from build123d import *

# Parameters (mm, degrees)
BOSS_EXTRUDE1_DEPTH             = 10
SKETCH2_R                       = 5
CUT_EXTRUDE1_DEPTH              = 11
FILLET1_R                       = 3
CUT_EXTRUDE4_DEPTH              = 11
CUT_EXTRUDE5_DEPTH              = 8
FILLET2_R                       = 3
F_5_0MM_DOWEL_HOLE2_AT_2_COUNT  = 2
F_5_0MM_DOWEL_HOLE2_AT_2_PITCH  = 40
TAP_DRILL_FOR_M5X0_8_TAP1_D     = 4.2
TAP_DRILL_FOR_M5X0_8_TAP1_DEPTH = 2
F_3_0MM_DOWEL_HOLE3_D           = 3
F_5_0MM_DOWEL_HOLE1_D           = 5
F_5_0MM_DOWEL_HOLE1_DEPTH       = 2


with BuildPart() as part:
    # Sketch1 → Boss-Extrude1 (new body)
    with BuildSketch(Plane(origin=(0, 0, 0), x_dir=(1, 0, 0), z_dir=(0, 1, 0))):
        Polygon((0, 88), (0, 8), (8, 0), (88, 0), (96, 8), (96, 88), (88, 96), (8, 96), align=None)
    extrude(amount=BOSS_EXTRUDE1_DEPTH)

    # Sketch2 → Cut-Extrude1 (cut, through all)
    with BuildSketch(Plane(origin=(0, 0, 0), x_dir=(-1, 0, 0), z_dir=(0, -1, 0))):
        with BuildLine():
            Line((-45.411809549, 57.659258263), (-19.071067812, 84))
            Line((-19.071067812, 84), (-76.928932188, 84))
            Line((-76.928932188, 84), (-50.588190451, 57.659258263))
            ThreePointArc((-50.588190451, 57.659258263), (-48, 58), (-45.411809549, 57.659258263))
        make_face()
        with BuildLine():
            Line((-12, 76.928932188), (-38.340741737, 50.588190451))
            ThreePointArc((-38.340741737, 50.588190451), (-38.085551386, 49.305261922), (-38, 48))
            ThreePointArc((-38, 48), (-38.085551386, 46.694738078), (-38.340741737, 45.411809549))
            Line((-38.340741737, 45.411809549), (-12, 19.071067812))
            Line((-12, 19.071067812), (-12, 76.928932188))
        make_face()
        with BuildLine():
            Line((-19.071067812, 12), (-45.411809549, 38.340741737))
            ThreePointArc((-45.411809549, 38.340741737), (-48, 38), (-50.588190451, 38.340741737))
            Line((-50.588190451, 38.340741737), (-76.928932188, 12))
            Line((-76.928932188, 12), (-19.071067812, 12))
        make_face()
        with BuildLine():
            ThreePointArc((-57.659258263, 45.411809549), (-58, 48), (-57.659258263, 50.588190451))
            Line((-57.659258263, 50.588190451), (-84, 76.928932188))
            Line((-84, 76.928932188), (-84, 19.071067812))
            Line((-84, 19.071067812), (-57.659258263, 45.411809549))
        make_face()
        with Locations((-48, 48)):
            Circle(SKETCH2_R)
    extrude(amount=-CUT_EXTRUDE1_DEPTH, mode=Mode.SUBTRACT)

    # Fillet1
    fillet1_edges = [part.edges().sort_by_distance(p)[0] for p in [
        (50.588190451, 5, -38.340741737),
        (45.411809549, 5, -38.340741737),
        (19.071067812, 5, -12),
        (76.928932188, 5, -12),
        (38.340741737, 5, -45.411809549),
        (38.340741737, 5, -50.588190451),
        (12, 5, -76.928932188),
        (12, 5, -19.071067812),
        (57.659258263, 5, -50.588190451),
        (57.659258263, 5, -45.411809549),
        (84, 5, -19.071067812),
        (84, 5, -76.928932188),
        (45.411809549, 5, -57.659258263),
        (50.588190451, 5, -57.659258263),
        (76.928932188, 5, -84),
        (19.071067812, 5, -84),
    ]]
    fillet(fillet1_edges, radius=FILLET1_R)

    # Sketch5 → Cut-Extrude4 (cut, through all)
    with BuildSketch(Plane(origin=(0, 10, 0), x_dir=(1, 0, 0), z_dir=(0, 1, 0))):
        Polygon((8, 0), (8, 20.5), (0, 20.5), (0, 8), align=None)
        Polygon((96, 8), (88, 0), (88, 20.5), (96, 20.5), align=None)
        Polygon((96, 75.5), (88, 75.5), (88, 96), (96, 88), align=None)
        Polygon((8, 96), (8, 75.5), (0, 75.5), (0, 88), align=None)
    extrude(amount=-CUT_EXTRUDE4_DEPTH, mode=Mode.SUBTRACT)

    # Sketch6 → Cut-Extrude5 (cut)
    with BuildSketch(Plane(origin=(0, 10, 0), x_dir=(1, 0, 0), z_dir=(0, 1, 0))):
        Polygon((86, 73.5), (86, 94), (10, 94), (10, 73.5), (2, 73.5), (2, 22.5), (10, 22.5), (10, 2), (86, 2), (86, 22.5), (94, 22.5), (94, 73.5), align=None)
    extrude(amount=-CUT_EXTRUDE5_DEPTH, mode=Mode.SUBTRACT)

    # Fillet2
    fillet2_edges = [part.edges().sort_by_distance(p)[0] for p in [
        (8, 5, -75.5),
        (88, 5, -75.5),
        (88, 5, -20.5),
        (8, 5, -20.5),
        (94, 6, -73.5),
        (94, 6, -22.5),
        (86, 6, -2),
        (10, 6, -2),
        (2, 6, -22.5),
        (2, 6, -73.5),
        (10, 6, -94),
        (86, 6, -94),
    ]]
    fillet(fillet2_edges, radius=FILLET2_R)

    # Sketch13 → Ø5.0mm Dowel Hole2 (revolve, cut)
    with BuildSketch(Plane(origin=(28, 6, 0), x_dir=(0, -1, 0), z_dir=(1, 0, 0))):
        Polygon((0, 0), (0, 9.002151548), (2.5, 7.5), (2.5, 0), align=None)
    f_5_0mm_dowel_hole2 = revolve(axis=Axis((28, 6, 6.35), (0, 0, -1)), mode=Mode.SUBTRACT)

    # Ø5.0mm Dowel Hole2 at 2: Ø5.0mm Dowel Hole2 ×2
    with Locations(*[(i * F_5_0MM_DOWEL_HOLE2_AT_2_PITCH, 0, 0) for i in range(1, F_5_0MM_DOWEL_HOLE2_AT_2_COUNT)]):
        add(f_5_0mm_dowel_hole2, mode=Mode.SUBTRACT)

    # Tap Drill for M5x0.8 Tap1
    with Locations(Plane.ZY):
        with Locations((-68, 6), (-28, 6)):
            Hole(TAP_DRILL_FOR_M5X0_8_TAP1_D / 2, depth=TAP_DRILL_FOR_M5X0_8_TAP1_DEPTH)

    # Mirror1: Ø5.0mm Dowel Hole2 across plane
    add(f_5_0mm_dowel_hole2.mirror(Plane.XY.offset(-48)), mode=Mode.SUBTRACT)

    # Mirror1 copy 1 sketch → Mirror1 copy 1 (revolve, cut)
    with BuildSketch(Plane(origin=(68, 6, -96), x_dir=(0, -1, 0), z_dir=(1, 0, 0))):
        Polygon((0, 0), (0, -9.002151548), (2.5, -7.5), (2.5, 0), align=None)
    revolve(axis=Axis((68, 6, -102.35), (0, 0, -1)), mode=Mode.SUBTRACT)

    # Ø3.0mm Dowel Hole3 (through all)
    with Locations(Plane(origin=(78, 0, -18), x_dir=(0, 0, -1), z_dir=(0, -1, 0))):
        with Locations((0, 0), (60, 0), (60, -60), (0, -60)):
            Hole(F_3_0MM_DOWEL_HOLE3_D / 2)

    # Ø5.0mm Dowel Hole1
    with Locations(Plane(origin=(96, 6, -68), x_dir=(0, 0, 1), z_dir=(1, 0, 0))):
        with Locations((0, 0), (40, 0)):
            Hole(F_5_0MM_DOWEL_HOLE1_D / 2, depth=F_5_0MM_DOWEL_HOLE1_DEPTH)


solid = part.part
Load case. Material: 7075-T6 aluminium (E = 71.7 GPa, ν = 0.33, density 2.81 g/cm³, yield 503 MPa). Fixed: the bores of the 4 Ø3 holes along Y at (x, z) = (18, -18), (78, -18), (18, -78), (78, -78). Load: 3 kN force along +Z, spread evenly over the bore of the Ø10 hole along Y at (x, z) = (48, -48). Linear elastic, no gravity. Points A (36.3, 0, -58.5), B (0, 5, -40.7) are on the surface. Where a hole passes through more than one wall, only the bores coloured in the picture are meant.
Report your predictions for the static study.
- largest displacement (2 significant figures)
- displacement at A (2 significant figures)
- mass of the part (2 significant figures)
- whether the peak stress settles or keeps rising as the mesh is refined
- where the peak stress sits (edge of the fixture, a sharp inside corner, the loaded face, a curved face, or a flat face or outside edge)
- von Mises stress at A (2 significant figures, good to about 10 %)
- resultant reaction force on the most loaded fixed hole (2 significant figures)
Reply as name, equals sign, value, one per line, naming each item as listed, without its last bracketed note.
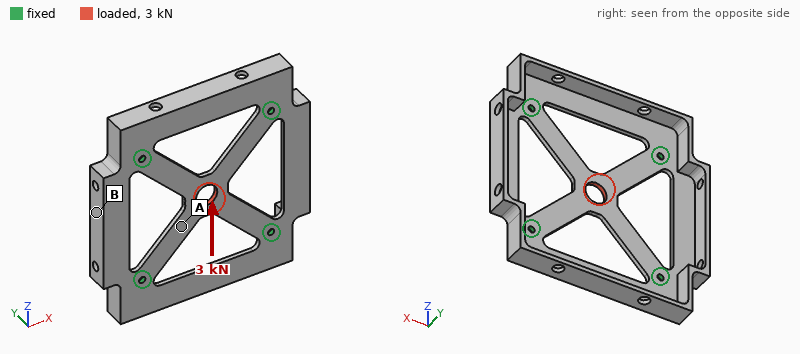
largest displacement = 43 µm
displacement at A = 28 µm
mass of the part = 46 g
whether the peak stress settles or keeps rising as the mesh is refined = keeps rising
where the peak stress sits = edge of the fixture
von Mises stress at A = 51 MPa
resultant reaction force on the most loaded fixed hole = 980 N
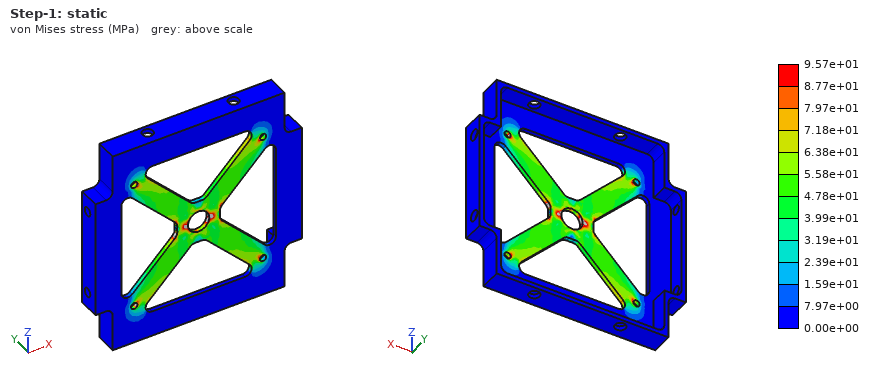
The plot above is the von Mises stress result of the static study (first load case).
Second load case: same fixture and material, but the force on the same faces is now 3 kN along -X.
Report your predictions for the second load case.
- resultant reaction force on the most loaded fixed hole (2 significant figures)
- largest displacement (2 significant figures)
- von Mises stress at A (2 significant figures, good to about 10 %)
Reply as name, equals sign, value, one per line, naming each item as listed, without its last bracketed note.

resultant reaction force on the most loaded fixed hole = 980 N
largest displacement = 43 µm
von Mises stress at A = 49 MPa
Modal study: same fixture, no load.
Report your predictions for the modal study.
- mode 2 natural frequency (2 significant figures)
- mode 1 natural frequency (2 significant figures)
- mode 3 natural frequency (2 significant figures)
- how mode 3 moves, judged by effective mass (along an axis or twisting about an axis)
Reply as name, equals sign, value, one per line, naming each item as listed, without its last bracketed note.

mode 2 natural frequency = 2300 Hz
mode 1 natural frequency = 1700 Hz
mode 3 natural frequency = 2500 Hz
how mode 3 moves, judged by effective mass = twisting about Z
